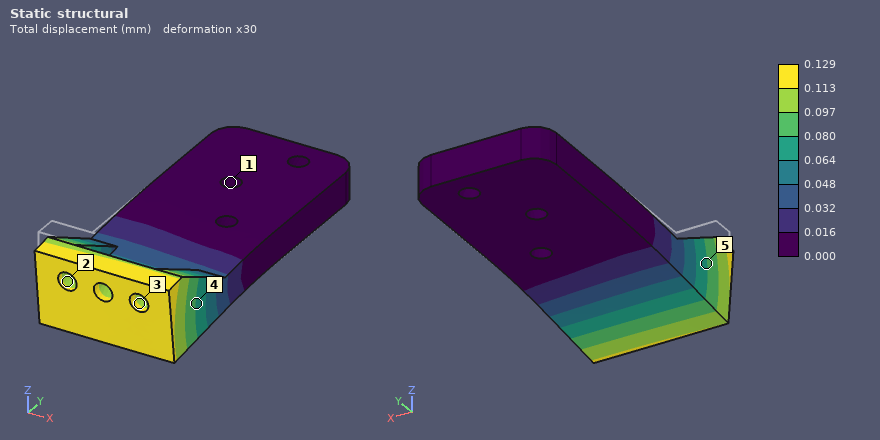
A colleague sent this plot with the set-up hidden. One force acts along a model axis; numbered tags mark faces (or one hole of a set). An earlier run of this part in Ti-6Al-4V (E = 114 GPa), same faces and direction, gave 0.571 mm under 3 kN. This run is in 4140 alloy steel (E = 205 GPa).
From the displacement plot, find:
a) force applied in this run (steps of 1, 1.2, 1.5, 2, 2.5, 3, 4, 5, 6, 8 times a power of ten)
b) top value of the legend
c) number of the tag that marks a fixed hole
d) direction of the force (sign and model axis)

1.2 kN
0.129 mm
1
-Z
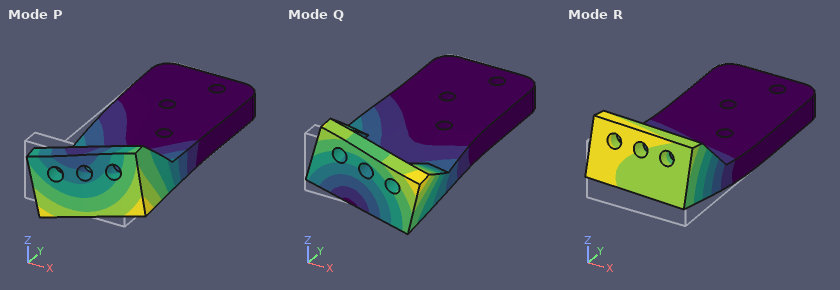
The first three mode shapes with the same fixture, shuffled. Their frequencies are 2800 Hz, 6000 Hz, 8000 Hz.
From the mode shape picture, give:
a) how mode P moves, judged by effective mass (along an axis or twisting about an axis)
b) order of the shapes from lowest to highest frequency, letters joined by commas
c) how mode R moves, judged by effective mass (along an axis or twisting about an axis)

along X
R, Q, P
along Z
